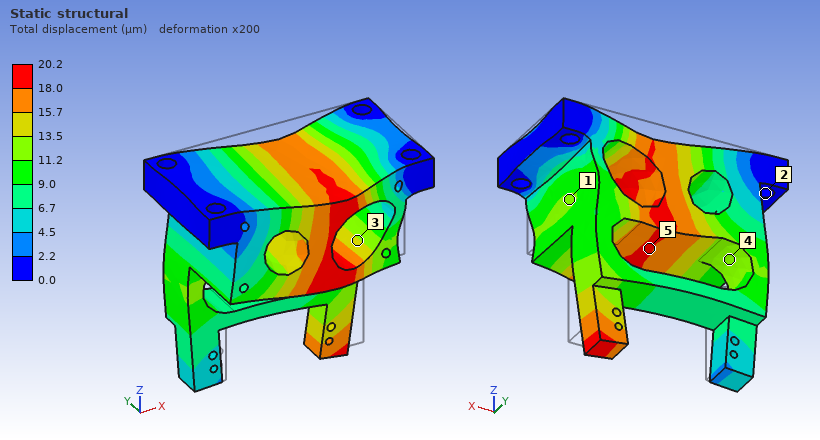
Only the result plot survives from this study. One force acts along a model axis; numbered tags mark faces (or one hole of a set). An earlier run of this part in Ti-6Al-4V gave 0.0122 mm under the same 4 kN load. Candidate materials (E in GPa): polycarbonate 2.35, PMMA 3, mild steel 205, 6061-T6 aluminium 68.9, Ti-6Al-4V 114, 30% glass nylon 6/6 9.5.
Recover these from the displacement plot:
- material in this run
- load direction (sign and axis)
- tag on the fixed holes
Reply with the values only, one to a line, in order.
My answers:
6061-T6 aluminium
-Z
2
